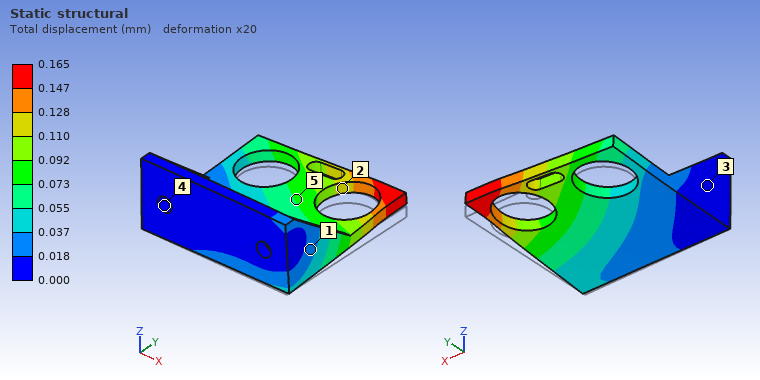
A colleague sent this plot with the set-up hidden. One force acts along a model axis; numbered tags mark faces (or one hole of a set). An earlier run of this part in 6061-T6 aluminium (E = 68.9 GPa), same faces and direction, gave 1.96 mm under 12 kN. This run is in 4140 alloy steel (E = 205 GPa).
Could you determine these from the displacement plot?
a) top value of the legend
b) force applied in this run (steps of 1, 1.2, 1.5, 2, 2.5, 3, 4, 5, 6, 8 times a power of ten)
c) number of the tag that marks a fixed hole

0.165 mm
3 kN
4
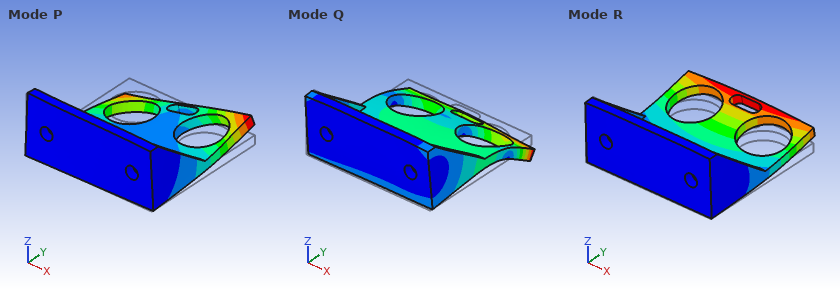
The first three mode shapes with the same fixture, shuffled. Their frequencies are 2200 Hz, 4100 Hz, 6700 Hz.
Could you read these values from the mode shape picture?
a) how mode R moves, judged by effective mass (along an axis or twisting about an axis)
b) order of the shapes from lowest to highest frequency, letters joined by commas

along Z
R, P, Q
